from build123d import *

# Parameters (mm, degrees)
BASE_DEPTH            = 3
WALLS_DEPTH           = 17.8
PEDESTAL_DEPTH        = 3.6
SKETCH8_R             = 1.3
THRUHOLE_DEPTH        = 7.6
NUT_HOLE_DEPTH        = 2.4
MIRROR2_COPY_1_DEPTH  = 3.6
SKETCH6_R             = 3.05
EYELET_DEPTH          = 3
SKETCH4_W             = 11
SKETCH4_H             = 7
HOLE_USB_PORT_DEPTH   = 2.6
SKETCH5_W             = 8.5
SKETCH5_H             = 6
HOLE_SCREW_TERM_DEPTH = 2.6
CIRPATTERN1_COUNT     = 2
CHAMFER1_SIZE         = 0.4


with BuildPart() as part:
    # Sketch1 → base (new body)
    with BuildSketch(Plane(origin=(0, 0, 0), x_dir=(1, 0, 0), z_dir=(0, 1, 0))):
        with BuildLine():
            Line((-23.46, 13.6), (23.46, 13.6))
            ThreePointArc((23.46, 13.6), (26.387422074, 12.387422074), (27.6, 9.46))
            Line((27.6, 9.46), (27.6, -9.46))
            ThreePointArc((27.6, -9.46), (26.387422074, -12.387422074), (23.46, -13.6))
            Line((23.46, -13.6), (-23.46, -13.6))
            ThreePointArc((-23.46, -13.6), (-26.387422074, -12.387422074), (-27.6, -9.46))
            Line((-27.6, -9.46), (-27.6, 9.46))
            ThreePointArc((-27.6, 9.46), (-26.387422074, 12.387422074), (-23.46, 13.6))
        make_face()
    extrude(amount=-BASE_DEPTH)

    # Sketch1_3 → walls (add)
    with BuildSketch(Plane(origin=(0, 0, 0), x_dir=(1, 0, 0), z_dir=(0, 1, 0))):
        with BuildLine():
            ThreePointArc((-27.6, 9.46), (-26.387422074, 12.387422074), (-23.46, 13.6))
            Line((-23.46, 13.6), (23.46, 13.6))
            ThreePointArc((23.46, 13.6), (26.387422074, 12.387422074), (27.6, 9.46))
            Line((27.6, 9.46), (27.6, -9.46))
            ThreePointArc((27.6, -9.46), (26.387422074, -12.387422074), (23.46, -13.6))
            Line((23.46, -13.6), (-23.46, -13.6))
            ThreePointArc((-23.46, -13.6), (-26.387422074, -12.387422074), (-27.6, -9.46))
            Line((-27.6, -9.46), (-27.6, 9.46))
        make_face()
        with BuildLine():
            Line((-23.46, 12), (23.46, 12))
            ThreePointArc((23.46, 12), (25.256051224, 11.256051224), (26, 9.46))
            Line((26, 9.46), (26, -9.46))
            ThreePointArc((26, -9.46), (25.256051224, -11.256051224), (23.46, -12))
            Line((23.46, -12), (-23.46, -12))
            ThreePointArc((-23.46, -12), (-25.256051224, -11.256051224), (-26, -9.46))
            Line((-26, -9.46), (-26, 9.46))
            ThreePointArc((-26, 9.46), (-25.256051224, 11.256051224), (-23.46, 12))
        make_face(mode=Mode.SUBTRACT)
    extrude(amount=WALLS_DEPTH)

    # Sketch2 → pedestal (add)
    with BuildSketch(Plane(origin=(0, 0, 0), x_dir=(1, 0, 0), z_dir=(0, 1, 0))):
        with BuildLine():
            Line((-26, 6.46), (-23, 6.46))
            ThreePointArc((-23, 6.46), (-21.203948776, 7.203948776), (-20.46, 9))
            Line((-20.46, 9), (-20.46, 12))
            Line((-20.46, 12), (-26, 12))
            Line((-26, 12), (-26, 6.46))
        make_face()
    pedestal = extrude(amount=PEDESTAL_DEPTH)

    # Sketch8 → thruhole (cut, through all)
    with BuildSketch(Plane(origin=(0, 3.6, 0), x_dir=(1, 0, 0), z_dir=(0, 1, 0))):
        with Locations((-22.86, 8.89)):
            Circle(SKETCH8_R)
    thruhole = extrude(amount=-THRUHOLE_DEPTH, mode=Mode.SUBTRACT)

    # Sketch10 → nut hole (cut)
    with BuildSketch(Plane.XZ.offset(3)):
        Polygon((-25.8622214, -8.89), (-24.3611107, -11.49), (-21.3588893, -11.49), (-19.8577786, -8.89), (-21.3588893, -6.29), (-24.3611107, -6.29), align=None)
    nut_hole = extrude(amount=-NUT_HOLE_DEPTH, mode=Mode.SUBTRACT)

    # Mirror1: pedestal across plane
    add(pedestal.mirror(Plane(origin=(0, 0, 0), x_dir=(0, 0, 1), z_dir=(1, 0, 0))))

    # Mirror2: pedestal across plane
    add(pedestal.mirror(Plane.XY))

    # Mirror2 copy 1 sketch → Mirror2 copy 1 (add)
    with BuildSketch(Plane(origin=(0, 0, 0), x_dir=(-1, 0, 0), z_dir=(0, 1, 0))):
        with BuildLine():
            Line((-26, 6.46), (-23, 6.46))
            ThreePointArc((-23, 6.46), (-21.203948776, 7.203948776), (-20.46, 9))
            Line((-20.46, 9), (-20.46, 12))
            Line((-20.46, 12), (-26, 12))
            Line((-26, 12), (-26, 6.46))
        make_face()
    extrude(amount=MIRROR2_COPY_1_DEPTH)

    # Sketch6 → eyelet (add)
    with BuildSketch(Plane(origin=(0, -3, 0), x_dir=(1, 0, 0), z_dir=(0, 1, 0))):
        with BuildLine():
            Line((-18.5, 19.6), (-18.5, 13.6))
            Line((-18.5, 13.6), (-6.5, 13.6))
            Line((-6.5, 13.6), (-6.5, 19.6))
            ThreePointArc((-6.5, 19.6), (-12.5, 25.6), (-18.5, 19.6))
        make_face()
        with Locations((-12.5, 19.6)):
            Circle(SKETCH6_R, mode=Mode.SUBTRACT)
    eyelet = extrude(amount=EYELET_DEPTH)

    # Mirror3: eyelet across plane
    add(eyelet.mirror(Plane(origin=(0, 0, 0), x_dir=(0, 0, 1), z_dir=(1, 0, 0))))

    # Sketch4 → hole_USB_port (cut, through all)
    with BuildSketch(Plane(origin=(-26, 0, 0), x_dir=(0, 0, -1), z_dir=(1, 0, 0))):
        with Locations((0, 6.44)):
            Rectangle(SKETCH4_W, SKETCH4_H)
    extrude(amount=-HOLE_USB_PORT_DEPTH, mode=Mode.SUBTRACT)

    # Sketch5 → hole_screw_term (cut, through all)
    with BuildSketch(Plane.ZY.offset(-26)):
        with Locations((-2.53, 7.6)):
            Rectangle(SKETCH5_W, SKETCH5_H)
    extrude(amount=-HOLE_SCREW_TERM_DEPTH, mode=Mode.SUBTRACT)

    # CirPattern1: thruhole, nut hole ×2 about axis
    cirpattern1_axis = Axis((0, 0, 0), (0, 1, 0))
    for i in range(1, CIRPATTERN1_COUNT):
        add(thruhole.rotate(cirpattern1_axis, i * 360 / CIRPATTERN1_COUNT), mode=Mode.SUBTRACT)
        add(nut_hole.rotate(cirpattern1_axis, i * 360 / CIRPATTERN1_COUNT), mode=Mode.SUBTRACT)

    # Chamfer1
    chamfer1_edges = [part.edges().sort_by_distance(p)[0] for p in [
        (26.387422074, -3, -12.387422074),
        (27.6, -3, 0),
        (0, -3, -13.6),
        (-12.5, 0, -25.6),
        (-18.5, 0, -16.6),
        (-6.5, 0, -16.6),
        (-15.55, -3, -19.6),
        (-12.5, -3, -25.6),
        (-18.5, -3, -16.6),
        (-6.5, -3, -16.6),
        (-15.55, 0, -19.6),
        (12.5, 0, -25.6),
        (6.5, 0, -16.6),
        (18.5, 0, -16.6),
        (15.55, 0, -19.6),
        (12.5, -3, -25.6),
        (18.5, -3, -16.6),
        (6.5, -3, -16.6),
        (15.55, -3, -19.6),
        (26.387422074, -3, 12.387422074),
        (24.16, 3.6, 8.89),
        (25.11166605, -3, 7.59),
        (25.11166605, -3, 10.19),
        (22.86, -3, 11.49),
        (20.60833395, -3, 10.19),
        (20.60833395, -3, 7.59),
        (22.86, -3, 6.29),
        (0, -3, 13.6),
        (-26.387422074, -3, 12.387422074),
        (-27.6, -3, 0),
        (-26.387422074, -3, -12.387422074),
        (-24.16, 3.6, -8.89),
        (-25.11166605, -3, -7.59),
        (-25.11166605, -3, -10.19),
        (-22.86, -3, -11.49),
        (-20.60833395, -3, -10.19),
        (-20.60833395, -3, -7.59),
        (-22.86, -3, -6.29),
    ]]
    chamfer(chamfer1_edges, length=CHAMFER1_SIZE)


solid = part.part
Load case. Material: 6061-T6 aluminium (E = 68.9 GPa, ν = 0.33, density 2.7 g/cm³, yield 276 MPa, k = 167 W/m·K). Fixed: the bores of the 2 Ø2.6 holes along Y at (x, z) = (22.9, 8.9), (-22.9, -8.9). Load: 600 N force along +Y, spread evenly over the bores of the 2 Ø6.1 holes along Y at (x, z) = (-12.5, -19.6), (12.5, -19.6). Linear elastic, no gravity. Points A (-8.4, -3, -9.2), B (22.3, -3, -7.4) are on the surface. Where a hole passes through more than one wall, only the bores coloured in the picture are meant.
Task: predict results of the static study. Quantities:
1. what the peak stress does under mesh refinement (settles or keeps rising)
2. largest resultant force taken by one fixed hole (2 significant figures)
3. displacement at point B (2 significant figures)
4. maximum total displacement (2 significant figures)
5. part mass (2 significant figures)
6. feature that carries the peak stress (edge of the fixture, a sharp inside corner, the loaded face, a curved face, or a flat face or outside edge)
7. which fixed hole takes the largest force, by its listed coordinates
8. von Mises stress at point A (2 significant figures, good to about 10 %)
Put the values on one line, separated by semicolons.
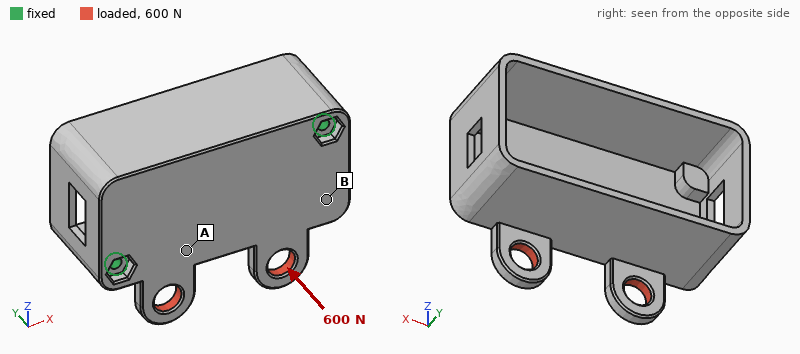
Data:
keeps rising; 500 N; 0.095 mm; 0.28 mm; 25 g; edge of the fixture; (-22.9, -8.9); 42 MPa
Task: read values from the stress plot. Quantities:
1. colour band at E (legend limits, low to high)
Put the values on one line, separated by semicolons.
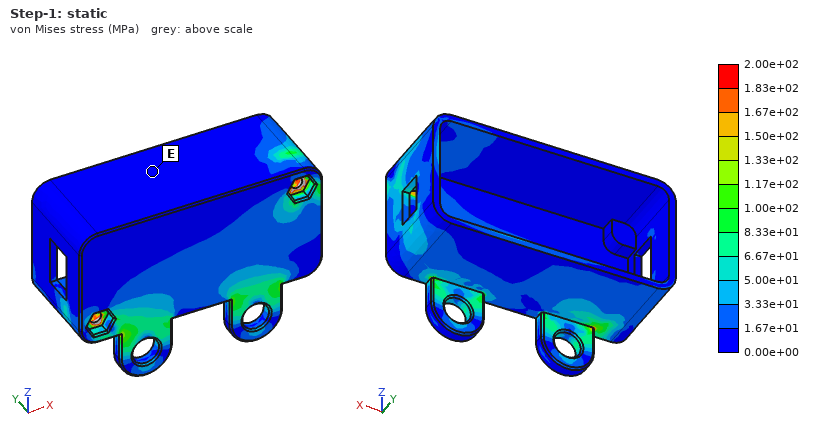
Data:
0.00e+00 to 1.67e+01 MPa
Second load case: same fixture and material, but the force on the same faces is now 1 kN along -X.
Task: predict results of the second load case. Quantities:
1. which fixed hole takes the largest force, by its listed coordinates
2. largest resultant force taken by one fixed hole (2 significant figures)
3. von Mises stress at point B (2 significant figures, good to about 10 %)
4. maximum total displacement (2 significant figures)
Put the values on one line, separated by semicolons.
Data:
(-22.9, -8.9); 800 N; 11 MPa; 33 µm
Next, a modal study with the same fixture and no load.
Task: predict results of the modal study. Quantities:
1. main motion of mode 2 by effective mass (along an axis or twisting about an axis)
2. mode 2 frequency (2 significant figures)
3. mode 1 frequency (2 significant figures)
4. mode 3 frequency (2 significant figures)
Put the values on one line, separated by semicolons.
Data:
along Y; 4300 Hz; 3500 Hz; 5100 Hz
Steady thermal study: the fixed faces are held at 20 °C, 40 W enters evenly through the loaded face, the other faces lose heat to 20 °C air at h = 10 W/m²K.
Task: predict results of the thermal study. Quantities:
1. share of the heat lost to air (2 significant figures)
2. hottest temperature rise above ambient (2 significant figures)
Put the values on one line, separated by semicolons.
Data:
4.9 %; 77 K
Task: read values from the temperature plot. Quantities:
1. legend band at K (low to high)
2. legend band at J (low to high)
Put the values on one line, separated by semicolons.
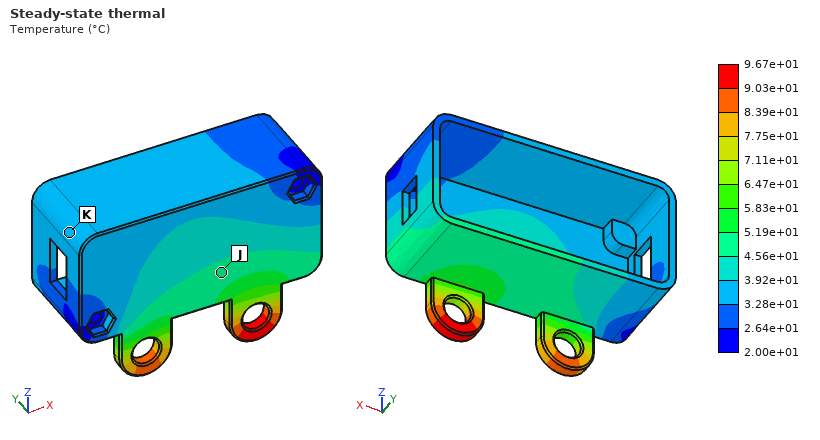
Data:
3.28e+01 to 3.92e+01 °C; 4.56e+01 to 5.19e+01 °C
